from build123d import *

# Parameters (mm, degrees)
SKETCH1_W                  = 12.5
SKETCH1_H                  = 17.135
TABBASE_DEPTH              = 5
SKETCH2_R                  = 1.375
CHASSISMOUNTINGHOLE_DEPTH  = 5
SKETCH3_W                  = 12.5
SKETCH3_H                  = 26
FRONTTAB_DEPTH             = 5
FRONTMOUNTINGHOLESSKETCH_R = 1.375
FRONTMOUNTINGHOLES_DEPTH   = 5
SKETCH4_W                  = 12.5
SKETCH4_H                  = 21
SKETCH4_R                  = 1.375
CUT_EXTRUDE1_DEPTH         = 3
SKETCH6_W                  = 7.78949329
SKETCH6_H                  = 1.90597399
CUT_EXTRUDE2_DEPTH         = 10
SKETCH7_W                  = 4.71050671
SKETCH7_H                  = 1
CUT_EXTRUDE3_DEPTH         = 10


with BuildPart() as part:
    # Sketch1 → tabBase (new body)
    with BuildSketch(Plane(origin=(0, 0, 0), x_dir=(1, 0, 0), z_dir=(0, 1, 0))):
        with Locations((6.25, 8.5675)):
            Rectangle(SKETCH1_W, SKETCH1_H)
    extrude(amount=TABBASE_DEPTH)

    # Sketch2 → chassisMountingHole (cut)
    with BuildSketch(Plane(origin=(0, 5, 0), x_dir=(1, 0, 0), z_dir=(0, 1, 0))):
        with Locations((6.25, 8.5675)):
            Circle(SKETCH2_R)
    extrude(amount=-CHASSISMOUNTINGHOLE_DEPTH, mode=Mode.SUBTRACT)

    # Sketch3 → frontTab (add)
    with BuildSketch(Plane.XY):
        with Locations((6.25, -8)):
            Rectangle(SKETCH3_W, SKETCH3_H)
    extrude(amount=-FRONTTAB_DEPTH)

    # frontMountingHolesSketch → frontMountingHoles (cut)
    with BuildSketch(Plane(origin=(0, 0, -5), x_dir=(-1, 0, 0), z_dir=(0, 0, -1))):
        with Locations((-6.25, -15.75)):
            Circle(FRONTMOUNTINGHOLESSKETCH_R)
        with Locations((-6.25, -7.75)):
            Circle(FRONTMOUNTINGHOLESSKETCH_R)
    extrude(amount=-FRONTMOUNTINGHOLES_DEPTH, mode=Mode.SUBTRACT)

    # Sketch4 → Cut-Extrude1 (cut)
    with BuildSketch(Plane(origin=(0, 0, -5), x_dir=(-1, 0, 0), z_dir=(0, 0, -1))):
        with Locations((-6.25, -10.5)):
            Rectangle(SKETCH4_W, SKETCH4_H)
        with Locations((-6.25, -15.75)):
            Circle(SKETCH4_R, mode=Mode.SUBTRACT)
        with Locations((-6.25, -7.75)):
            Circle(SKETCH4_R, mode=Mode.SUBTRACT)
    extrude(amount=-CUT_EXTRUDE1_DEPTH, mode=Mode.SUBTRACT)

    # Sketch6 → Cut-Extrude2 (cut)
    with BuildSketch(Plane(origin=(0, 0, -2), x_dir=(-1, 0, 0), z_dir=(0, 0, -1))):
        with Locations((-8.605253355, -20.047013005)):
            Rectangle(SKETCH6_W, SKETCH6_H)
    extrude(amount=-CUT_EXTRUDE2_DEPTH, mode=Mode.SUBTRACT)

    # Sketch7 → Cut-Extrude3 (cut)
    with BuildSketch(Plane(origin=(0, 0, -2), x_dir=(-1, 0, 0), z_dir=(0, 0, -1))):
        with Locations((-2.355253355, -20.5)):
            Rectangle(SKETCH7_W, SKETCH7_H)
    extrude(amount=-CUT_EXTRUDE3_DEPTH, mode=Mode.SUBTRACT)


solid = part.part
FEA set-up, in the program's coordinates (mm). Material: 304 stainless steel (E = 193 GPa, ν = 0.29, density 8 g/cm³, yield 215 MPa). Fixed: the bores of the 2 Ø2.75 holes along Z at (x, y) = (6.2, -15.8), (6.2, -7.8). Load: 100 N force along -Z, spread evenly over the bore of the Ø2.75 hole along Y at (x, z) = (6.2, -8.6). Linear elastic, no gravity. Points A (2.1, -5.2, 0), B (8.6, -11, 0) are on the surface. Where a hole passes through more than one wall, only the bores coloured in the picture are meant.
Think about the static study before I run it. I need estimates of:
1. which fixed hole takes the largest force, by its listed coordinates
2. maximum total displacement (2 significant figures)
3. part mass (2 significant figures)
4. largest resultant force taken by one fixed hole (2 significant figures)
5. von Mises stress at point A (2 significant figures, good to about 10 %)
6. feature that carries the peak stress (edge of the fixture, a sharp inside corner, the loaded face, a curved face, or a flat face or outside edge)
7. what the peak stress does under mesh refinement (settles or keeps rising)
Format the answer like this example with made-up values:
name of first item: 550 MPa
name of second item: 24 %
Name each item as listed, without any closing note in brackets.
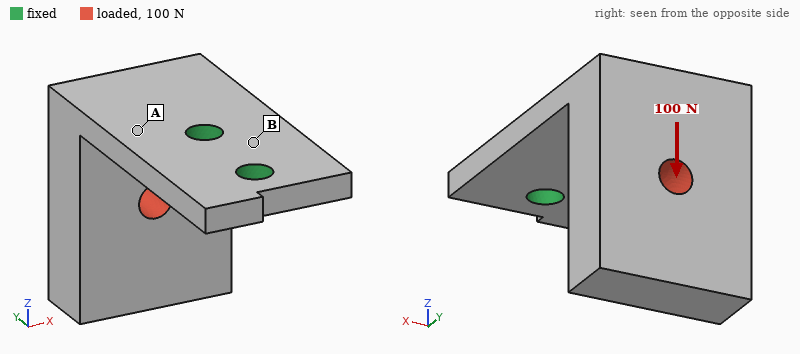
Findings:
which fixed hole takes the largest force, by its listed coordinates: (6.2, -7.8)
maximum total displacement: 55 µm
part mass: 12 g
largest resultant force taken by one fixed hole: 130 N
von Mises stress at point A: 72 MPa
feature that carries the peak stress: edge of the fixture
what the peak stress does under mesh refinement: keeps rising
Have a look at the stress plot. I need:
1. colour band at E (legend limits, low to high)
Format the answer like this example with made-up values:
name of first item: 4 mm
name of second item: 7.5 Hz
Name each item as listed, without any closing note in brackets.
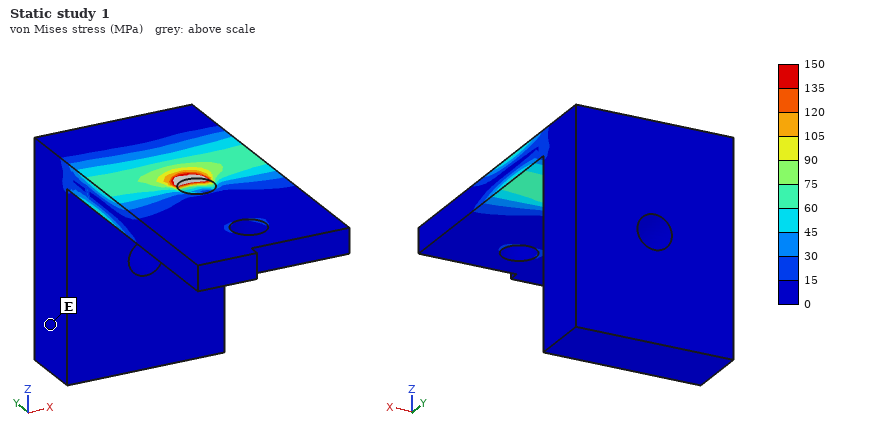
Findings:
colour band at E: 0 to 15 MPa
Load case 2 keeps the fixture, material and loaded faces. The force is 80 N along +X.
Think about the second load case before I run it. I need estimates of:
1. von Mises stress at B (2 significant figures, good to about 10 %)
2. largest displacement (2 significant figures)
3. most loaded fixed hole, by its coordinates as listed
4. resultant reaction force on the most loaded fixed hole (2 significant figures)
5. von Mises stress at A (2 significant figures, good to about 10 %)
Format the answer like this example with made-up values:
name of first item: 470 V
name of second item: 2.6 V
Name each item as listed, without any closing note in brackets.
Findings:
von Mises stress at B: 19 MPa
largest displacement: 28 µm
most loaded fixed hole, by its coordinates as listed: (6.2, -7.8)
resultant reaction force on the most loaded fixed hole: 140 N
von Mises stress at A: 35 MPa
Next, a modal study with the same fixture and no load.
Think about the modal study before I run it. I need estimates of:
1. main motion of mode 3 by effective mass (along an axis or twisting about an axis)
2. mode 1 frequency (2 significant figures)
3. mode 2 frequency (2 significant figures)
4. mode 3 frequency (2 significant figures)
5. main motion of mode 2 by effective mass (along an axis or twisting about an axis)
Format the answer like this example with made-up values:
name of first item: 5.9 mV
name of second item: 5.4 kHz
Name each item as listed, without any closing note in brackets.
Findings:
main motion of mode 3 by effective mass: along Z
mode 1 frequency: 2200 Hz
mode 2 frequency: 3400 Hz
mode 3 frequency: 9800 Hz
main motion of mode 2 by effective mass: along X
